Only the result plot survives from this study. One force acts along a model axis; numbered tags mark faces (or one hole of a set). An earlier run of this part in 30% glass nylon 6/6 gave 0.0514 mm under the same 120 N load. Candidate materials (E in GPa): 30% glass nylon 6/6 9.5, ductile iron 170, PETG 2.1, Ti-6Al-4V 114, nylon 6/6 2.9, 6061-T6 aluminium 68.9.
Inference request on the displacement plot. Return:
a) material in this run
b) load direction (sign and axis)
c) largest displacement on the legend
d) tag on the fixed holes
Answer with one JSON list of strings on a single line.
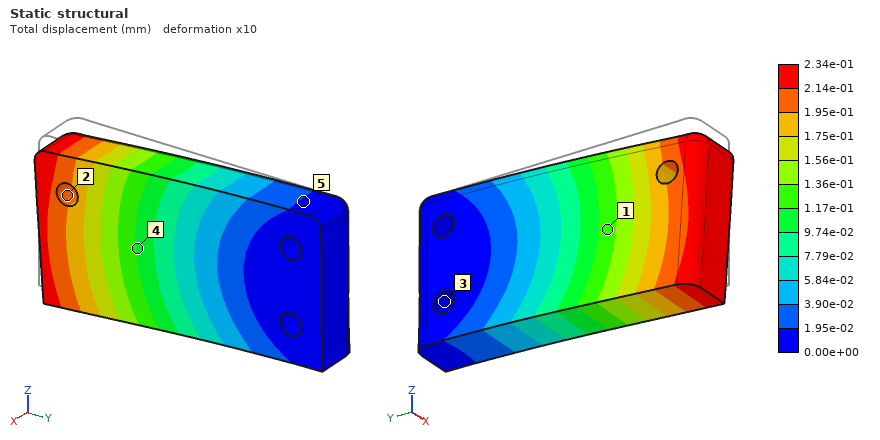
["PETG", "-Z", "2.34e-01 mm", "3"]
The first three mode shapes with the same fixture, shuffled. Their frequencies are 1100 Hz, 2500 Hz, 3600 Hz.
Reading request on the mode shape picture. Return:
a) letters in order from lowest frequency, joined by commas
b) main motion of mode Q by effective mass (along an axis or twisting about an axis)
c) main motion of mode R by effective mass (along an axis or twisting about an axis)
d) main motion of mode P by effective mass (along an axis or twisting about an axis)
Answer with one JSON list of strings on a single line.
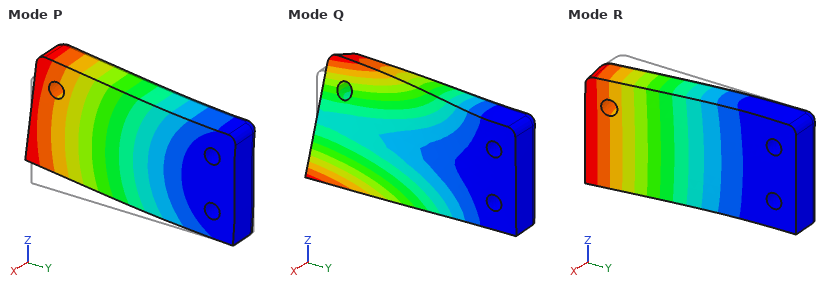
["R, P, Q", "twisting about Y", "along X", "along Z"]
